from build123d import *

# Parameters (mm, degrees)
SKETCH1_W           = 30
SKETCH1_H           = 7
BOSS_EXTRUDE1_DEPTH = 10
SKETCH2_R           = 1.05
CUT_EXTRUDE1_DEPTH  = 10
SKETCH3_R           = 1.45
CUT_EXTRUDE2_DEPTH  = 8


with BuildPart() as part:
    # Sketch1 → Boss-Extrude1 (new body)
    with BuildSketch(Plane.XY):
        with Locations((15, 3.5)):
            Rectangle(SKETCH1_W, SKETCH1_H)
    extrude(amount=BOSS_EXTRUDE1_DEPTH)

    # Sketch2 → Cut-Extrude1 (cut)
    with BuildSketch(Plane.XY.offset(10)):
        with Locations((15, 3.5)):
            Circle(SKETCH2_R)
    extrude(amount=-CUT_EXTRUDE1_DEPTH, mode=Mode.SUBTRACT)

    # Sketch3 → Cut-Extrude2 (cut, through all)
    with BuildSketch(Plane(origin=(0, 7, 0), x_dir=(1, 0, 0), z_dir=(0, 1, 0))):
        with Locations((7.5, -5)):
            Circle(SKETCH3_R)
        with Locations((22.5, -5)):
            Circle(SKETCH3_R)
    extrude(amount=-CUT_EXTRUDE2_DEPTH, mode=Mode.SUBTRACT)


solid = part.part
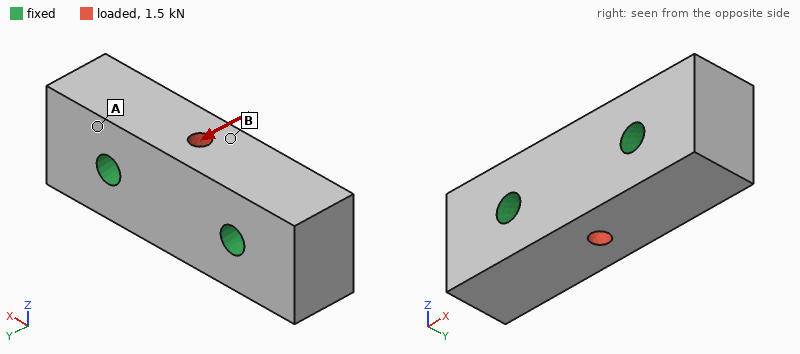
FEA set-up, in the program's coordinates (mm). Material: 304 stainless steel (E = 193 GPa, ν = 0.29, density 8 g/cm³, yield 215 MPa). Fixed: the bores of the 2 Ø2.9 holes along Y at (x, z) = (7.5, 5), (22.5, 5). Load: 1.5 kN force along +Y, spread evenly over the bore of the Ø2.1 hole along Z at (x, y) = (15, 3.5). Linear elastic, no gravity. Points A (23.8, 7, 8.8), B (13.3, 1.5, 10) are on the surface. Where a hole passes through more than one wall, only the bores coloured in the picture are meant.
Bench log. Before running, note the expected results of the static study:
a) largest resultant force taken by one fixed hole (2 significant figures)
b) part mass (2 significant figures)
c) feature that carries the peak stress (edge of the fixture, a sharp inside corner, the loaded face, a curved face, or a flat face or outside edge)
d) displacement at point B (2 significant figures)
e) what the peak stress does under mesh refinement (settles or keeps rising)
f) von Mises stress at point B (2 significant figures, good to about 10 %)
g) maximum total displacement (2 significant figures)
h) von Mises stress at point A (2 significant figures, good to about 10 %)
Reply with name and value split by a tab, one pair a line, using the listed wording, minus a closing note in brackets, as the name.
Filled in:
largest resultant force taken by one fixed hole	750 N
part mass	16 g
feature that carries the peak stress	edge of the fixture
displacement at point B	1.4 µm
what the peak stress does under mesh refinement	keeps rising
von Mises stress at point B	22 MPa
maximum total displacement	1.8 µm
von Mises stress at point A	8.8 MPa
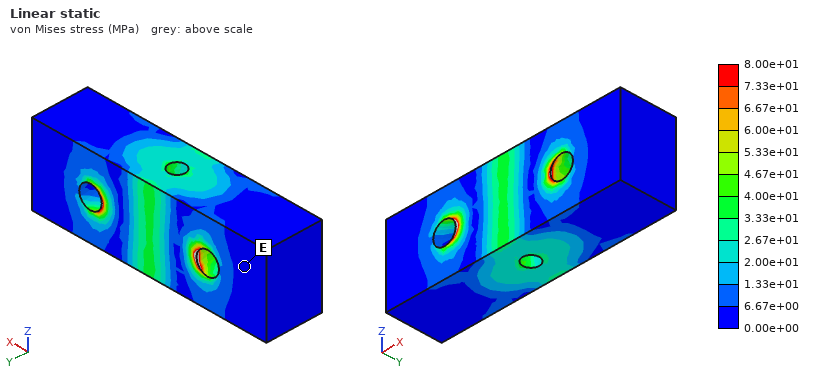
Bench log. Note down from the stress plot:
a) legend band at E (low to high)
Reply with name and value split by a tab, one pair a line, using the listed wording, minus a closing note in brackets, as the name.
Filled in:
legend band at E	0.00e+00 to 6.67e+00 MPa
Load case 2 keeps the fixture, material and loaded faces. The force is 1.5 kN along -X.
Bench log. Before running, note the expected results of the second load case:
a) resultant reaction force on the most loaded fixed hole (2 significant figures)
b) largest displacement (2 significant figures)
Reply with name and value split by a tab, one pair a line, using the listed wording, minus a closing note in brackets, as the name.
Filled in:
resultant reaction force on the most loaded fixed hole	750 N
largest displacement	0.56 µm
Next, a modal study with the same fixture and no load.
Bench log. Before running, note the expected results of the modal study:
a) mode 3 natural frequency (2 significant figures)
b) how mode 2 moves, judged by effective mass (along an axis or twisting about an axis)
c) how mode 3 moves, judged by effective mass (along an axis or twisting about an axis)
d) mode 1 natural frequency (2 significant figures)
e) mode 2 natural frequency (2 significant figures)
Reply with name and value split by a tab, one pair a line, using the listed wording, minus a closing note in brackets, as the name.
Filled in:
mode 3 natural frequency	67 kHz
how mode 2 moves, judged by effective mass	twisting about Y
how mode 3 moves, judged by effective mass	along Y
mode 1 natural frequency	57 kHz
mode 2 natural frequency	61 kHz
